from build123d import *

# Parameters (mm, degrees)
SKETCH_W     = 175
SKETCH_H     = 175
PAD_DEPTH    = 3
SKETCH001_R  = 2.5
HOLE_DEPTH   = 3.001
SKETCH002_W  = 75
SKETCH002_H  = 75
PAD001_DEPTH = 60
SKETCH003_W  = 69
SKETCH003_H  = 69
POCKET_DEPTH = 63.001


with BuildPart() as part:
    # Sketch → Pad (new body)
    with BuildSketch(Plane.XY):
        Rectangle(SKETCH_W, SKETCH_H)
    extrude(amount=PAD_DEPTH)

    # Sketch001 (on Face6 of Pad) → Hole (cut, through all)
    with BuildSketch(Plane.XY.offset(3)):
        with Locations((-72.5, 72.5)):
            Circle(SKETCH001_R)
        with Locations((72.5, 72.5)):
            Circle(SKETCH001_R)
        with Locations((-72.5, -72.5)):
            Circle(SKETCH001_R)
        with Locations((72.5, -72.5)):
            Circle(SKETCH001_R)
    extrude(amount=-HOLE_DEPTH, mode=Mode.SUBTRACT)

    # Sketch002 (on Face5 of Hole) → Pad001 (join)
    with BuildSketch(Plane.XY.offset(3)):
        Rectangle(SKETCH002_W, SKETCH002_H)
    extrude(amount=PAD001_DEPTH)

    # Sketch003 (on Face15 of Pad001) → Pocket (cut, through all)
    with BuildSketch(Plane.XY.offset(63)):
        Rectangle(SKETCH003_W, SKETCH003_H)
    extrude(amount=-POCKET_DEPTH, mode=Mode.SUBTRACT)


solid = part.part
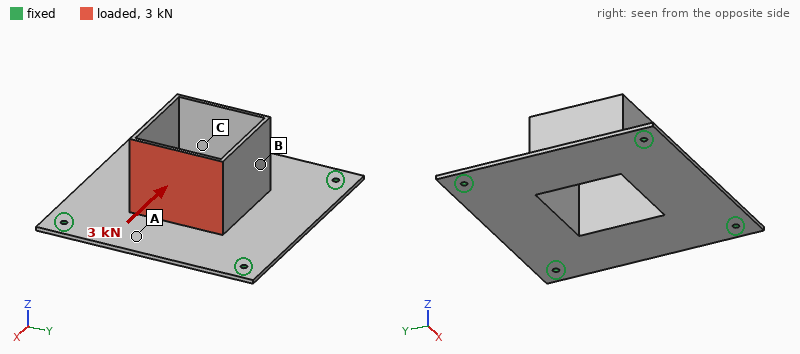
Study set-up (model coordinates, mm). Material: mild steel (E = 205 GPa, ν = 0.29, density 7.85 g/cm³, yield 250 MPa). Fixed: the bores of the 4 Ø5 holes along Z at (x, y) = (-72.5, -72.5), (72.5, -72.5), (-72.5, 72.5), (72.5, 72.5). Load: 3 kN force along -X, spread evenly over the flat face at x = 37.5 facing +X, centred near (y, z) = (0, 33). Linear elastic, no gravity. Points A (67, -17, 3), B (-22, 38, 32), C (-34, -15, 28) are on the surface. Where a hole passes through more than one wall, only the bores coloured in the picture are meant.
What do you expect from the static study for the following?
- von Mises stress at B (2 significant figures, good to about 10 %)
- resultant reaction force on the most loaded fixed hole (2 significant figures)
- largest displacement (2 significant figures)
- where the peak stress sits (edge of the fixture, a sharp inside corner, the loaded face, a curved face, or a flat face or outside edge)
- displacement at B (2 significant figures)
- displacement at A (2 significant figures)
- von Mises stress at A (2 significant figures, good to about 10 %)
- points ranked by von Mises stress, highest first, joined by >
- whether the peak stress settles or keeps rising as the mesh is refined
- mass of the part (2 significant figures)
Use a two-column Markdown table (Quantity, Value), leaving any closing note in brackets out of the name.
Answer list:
| Quantity | Value |
|---|---|
| von Mises stress at B | 23 MPa |
| resultant reaction force on the most loaded fixed hole | 940 N |
| largest displacement | 0.48 mm |
| where the peak stress sits | edge of the fixture |
| displacement at B | 0.16 mm |
| displacement at A | 0.21 mm |
| von Mises stress at A | 44 MPa |
| points ranked by von Mises stress, highest first, joined by > | A > B > C |
| whether the peak stress settles or keeps rising as the mesh is refined | keeps rising |
| mass of the part | 1.0 kg |
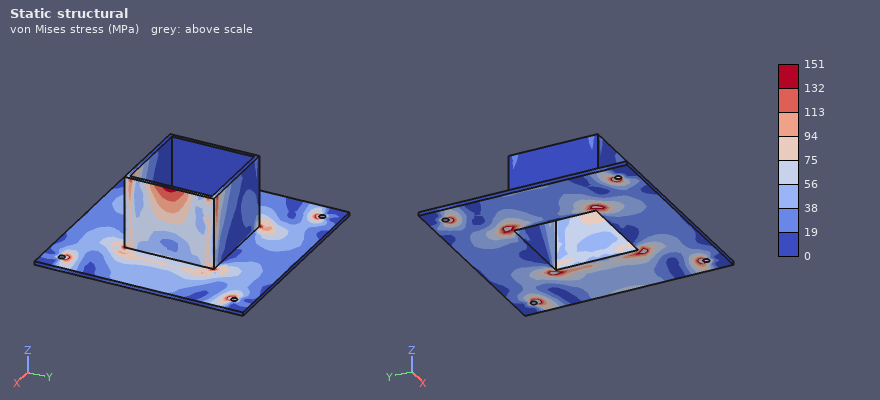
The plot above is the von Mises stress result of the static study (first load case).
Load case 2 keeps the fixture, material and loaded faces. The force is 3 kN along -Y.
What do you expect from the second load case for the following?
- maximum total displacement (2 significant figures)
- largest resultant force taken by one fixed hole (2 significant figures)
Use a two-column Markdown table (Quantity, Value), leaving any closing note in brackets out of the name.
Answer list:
| Quantity | Value |
|---|---|
| maximum total displacement | 0.40 mm |
| largest resultant force taken by one fixed hole | 1.3 kN |
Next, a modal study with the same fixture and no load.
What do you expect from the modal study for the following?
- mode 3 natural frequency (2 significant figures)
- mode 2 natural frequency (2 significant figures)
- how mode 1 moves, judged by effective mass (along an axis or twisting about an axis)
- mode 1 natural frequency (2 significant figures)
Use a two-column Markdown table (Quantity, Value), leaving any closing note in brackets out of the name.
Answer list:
| Quantity | Value |
|---|---|
| mode 3 natural frequency | 650 Hz |
| mode 2 natural frequency | 650 Hz |
| how mode 1 moves, judged by effective mass | along Z |
| mode 1 natural frequency | 490 Hz |
